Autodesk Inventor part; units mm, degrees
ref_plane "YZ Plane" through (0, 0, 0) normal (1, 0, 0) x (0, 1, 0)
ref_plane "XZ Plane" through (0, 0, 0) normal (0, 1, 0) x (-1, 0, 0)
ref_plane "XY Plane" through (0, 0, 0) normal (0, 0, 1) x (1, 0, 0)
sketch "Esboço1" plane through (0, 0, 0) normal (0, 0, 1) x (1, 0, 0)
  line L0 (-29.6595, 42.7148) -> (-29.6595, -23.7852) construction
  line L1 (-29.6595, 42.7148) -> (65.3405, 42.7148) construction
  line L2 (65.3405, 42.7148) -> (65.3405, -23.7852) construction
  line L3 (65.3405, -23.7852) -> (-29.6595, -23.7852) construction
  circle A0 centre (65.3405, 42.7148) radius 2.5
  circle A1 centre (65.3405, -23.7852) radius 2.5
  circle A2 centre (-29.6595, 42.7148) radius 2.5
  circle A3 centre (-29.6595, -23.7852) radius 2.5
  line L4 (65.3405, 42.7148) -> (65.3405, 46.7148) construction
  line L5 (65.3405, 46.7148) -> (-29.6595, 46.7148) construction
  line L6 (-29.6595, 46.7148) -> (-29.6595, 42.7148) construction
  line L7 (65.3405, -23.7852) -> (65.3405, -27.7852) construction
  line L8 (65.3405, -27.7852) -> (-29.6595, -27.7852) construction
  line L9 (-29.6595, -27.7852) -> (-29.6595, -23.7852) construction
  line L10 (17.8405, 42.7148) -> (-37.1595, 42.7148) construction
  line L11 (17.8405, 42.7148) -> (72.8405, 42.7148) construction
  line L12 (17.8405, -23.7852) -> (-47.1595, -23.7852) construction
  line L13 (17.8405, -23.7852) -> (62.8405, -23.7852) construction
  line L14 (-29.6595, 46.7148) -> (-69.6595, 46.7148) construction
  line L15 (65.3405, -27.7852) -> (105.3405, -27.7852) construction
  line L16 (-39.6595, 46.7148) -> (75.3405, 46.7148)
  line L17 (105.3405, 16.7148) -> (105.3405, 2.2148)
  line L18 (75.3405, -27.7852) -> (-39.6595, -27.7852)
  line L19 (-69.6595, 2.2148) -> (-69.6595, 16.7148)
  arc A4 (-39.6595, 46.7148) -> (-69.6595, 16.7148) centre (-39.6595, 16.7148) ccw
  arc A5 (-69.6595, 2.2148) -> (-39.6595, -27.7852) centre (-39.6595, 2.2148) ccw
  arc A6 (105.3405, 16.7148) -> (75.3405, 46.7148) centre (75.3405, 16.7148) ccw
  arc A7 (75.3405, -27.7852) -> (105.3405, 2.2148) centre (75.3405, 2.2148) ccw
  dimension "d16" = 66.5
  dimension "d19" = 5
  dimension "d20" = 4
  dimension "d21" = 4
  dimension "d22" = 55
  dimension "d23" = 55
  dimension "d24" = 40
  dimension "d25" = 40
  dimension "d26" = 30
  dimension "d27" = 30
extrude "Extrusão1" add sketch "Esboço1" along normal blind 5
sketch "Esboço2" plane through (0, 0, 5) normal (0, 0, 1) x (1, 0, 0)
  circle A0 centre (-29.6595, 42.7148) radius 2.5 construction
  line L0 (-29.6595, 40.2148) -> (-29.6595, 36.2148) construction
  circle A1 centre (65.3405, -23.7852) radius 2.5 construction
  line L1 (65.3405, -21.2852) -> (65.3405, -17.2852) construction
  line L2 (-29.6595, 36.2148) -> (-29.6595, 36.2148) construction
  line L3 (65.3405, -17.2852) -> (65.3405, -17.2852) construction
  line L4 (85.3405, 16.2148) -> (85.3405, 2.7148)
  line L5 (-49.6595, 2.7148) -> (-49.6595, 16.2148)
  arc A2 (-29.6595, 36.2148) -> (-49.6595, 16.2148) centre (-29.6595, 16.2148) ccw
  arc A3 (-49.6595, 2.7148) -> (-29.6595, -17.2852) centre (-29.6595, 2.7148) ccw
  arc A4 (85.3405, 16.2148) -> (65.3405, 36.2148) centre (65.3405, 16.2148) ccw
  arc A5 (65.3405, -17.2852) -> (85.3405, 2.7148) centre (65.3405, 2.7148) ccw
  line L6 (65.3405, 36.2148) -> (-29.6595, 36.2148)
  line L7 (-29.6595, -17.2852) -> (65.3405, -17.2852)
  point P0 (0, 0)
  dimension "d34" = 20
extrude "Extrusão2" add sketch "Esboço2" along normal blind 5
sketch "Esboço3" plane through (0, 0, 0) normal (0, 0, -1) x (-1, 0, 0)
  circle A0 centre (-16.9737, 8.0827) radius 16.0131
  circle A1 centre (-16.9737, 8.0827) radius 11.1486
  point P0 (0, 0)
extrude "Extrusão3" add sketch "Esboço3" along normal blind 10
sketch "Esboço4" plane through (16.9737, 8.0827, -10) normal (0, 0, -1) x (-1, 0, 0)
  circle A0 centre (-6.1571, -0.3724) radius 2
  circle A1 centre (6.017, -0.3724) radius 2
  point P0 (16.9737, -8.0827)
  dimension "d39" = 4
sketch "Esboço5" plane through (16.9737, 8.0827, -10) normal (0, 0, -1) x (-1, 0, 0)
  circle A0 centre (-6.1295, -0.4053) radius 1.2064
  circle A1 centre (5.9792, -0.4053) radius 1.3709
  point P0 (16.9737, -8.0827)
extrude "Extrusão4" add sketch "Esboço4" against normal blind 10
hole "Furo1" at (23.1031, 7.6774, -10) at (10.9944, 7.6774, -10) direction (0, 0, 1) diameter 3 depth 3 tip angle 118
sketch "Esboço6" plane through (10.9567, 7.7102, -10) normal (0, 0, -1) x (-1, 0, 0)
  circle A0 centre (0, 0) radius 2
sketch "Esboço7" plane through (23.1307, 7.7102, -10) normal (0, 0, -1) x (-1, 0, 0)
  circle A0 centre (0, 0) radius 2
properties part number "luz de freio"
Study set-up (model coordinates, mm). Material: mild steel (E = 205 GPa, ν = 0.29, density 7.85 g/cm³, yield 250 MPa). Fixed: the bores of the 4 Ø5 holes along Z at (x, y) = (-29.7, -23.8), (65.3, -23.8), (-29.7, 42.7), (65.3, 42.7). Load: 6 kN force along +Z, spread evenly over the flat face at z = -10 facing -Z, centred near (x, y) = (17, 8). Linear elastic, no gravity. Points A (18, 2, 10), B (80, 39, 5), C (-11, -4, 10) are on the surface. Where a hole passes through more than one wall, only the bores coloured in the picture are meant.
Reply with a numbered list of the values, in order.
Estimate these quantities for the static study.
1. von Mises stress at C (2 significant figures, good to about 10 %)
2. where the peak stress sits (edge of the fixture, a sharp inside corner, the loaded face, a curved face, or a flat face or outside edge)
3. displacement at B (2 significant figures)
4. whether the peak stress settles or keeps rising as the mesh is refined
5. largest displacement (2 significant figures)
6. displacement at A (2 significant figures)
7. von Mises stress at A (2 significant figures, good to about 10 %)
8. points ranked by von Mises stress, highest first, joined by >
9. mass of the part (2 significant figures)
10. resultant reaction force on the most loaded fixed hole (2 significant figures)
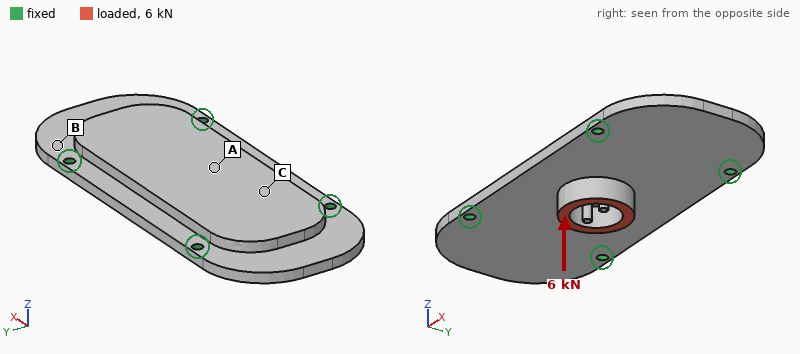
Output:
1. 29 MPa
2. edge of the fixture
3. 9.2 µm
4. keeps rising
5. 56 µm
6. 54 µm
7. 57 MPa
8. A > C > B
9. 780 g
10. 2.6 kN
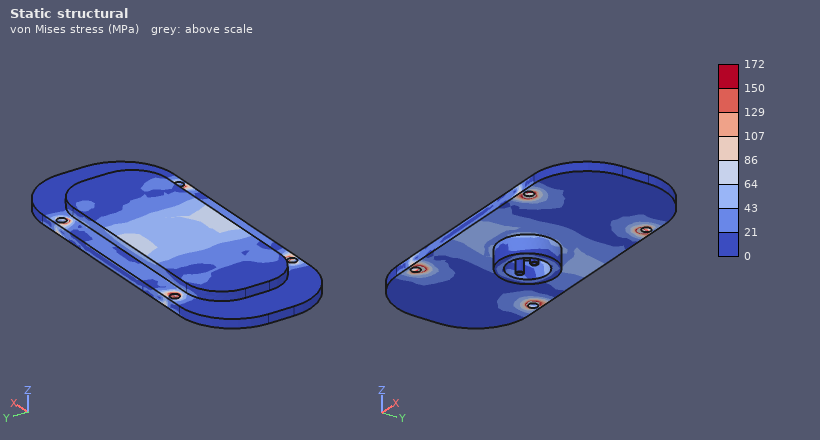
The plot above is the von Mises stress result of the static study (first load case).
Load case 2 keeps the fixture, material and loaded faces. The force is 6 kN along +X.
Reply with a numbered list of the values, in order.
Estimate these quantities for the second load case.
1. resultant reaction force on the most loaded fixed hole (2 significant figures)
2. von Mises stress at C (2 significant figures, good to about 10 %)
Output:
1. 1.6 kN
2. 13 MPa
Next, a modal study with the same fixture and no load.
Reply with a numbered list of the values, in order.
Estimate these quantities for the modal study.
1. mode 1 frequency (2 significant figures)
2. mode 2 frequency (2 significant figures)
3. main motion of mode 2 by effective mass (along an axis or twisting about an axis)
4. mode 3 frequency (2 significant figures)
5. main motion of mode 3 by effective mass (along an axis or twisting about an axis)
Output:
1. 2900 Hz
2. 3700 Hz
3. twisting about Y
4. 3900 Hz
5. along Z
